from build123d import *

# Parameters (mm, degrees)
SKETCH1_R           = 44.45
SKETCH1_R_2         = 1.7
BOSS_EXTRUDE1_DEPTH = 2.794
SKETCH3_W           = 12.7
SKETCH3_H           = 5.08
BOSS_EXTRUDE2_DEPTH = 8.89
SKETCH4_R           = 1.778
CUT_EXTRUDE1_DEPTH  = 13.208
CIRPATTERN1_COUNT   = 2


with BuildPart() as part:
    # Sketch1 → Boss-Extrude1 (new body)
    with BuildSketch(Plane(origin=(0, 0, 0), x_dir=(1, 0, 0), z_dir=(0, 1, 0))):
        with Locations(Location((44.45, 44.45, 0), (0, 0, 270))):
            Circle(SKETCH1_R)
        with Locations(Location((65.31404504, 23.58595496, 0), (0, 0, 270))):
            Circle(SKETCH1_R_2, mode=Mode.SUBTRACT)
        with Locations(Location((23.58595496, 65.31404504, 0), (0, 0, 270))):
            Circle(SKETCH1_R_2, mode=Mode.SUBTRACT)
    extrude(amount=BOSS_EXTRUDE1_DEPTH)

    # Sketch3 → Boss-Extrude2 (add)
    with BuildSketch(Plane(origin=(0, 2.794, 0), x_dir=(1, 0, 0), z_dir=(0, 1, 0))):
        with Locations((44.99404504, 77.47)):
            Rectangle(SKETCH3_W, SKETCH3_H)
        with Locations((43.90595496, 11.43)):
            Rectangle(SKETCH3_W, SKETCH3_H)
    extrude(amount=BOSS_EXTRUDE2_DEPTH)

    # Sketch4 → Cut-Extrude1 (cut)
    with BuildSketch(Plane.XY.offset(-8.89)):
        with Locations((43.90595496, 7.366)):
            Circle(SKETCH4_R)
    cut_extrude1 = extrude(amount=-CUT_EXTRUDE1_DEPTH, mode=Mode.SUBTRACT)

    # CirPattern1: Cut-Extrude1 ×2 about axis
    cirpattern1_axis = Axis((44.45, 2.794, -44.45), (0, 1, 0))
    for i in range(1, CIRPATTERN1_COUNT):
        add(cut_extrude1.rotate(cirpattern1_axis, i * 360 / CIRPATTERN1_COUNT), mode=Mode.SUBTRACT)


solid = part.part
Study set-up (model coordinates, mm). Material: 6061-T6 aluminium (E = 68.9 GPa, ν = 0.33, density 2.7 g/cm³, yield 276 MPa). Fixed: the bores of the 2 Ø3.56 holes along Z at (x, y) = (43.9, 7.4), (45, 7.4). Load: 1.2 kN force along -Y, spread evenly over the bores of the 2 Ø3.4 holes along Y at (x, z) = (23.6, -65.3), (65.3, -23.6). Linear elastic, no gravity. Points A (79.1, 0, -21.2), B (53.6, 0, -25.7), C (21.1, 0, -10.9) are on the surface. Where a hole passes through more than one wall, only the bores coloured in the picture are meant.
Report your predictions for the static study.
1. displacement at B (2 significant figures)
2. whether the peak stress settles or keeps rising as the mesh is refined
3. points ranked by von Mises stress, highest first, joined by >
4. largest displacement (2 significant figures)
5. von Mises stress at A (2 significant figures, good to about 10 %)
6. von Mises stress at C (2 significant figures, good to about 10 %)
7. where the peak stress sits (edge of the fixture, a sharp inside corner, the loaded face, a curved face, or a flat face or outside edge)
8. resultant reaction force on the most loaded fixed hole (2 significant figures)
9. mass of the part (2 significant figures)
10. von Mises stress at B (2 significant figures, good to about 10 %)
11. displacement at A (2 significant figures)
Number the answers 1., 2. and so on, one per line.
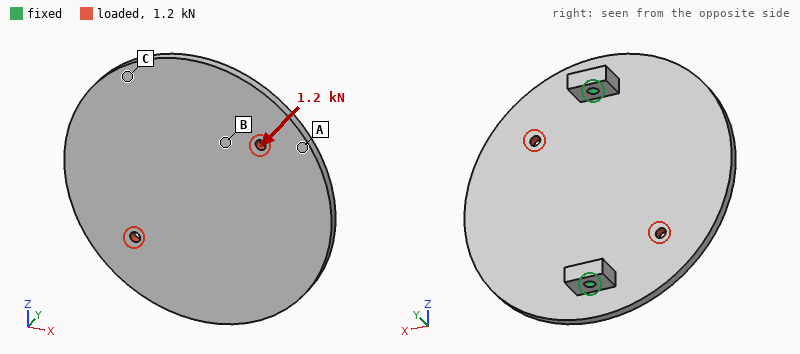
1. 0.14 mm
2. keeps rising
3. B > A > C
4. 0.57 mm
5. 63 MPa
6. 33 MPa
7. a sharp inside corner
8. 900 N
9. 50 g
10. 95 MPa
11. 0.49 mm
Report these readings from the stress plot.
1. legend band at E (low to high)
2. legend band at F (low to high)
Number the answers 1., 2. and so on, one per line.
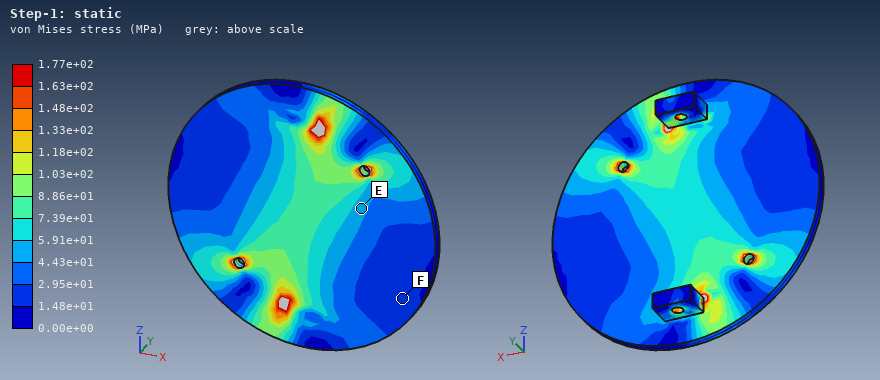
1. 4.43e+01 to 5.91e+01 MPa
2. 1.48e+01 to 2.95e+01 MPa
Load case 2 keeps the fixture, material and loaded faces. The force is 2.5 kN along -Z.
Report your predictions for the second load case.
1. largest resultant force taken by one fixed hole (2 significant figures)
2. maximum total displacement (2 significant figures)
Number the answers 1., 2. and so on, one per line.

1. 1.3 kN
2. 24 µm
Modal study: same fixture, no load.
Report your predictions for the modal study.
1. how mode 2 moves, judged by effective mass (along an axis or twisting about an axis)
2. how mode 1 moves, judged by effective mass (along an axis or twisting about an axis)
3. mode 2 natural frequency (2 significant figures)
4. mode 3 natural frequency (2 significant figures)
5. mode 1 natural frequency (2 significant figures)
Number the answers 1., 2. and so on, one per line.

1. along Y
2. twisting about Z
3. 1500 Hz
4. 3200 Hz
5. 1200 Hz
